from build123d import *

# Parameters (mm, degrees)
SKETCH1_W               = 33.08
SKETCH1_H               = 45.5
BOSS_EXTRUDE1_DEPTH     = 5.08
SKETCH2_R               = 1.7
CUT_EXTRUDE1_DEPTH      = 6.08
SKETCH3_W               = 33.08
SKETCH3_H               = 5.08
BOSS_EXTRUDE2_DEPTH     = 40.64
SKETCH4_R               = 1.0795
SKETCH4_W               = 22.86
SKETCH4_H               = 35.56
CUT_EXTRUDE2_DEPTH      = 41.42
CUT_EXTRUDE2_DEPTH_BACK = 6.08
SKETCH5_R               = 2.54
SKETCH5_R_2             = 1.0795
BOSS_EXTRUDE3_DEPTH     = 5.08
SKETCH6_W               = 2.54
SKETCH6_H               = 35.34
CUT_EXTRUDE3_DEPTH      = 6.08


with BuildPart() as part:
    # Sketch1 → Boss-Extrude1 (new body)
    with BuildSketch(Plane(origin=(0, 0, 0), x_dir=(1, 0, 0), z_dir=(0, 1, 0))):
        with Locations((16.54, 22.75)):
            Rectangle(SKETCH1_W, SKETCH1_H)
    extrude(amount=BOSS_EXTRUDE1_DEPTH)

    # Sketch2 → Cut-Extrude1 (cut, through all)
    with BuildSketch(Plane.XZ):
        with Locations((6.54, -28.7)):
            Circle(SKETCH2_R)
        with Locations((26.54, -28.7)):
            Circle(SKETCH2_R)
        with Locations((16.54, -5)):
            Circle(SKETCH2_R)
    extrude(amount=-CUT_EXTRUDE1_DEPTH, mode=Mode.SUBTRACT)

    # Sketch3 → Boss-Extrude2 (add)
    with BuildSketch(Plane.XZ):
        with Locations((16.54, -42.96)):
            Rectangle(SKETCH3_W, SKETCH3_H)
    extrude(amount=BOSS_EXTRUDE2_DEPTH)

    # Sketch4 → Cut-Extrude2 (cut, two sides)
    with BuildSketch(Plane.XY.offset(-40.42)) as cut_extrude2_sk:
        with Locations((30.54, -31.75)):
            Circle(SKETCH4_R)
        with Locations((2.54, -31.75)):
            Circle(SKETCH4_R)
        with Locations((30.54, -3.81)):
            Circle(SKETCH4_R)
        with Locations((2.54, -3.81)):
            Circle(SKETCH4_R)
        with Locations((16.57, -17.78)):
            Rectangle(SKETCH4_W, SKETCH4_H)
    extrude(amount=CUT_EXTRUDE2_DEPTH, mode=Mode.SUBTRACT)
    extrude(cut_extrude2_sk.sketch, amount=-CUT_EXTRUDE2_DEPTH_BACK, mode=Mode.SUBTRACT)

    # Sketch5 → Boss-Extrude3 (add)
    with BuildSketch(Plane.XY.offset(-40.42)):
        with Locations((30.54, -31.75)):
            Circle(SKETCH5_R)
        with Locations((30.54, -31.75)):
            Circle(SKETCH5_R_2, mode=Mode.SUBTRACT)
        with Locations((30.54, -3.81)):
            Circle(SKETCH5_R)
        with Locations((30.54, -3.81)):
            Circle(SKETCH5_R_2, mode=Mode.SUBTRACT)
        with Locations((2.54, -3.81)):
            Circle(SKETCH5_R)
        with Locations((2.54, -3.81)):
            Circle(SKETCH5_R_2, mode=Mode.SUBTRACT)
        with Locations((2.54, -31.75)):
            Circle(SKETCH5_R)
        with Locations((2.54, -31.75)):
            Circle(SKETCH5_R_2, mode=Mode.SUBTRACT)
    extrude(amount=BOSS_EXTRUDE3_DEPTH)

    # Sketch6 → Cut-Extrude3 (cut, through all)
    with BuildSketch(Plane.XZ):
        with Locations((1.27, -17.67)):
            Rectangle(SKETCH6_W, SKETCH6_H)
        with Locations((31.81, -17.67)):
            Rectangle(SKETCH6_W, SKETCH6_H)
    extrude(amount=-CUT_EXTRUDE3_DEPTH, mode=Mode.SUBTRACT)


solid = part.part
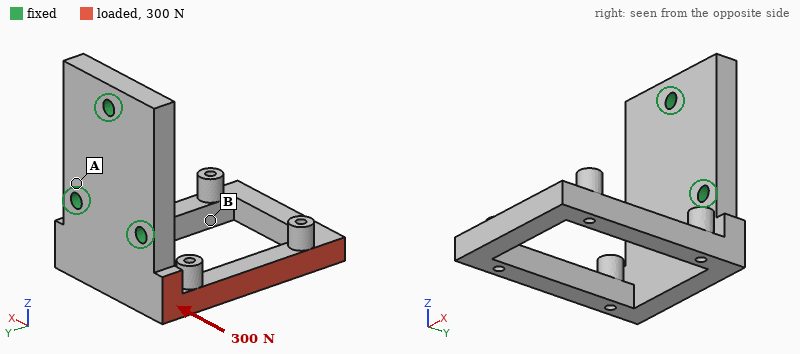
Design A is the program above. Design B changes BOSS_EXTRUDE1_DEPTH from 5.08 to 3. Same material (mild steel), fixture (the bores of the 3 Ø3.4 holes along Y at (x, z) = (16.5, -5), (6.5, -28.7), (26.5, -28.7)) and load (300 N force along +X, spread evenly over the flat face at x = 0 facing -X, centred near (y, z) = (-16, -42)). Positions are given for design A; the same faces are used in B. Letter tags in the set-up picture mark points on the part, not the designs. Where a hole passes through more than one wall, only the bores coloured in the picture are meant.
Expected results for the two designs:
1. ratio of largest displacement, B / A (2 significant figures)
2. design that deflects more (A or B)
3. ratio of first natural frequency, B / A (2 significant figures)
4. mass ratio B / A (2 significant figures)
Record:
2.1
B
0.69
0.72
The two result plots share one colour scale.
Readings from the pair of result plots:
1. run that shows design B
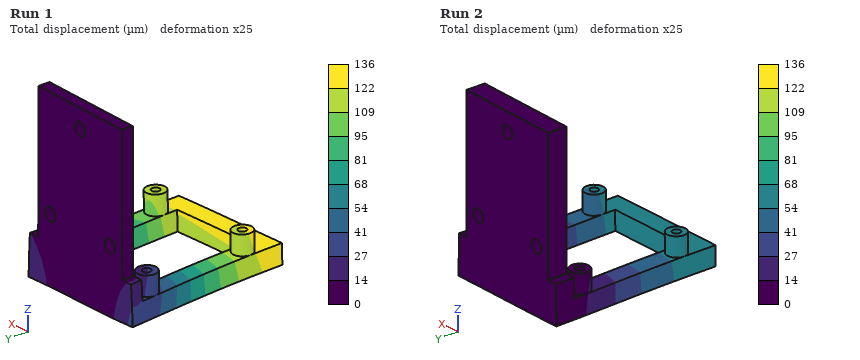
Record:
Run 1
